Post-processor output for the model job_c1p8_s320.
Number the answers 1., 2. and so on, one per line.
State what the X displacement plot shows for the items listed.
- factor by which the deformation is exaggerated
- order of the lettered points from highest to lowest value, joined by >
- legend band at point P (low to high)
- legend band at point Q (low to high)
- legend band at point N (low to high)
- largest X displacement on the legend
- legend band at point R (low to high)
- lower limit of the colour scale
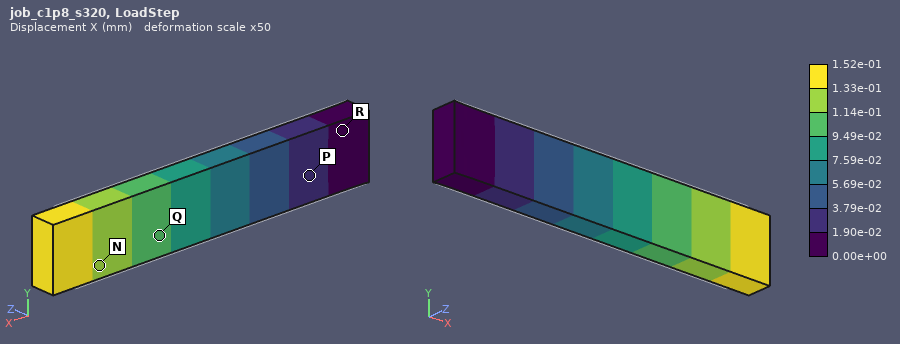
1. 50
2. N > Q > P > R
3. 1.90e-02 to 3.79e-02 mm
4. 9.49e-02 to 1.14e-01 mm
5. 1.14e-01 to 1.33e-01 mm
6. 1.52e-01 mm
7. 0.00e+00 to 1.90e-02 mm
8. 0.00e+00 mm
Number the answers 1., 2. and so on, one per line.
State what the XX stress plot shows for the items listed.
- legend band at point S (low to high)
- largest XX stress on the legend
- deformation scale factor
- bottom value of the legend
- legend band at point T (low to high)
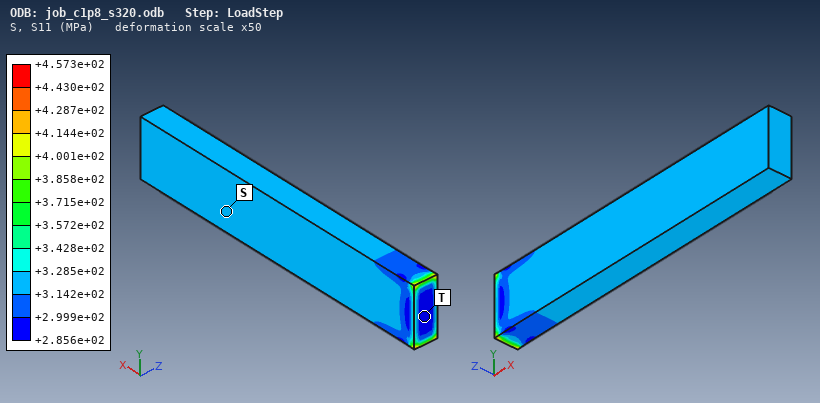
1. +3.142e+02 to +3.285e+02 MPa
2. +4.573e+02 MPa
3. 50
4. +2.856e+02 MPa
5. +2.856e+02 to +2.999e+02 MPa
